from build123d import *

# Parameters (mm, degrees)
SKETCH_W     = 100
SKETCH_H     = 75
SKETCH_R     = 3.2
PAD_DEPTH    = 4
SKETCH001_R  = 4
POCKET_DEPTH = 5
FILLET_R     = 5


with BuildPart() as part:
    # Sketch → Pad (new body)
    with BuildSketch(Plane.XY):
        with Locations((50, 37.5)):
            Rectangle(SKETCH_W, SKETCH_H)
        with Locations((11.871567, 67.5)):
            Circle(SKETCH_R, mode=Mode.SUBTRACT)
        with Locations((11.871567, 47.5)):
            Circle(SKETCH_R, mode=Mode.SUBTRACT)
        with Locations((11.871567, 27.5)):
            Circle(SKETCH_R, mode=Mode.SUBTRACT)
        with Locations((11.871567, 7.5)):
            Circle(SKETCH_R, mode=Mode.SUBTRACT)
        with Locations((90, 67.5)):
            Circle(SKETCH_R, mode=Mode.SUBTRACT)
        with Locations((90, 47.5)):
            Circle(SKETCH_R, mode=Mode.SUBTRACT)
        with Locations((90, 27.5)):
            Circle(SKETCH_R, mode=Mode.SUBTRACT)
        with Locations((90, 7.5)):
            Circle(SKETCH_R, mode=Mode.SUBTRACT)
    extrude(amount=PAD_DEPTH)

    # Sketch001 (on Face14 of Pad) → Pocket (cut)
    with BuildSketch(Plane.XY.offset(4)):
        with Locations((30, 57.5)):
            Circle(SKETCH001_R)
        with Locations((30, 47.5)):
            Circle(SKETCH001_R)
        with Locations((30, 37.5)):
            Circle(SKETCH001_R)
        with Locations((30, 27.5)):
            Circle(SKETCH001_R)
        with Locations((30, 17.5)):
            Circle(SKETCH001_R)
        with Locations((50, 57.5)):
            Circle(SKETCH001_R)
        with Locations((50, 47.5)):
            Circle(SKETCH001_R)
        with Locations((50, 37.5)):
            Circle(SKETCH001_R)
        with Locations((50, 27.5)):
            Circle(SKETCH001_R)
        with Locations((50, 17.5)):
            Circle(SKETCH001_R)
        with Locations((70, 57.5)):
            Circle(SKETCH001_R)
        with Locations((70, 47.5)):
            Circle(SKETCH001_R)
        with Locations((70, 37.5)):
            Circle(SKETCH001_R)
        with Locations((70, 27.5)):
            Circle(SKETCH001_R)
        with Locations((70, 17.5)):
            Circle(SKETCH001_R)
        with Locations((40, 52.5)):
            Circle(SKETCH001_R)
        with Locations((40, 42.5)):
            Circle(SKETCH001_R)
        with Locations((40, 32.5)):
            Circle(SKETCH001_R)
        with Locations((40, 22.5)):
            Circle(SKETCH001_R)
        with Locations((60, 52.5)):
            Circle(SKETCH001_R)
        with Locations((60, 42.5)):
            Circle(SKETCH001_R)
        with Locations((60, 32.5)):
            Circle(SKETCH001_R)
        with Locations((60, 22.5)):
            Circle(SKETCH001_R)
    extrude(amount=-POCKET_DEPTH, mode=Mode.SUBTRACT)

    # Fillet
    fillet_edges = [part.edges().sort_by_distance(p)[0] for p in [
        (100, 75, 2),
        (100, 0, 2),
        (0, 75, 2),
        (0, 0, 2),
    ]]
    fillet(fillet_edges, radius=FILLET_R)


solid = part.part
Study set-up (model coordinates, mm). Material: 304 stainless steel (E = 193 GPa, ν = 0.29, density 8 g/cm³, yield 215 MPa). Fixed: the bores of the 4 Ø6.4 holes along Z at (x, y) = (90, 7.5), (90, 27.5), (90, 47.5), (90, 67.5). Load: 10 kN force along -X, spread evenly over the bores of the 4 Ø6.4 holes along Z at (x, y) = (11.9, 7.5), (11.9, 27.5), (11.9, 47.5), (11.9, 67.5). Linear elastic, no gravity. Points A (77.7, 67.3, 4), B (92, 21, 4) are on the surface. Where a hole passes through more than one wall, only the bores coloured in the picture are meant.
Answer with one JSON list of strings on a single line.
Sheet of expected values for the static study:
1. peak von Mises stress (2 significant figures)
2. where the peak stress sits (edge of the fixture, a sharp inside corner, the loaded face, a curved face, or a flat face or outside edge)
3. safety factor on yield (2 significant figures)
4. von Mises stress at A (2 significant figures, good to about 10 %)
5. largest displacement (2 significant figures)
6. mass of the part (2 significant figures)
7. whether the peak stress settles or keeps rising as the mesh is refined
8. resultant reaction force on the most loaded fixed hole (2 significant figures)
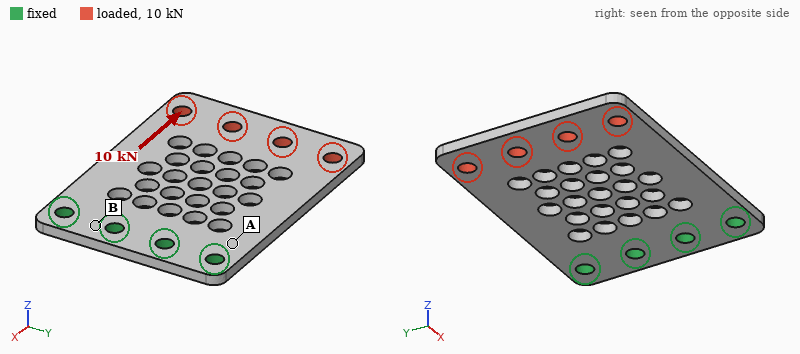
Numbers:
["150 MPa", "a curved face", "1.4", "64 MPa", "28 µm", "190 g", "settles", "3.5 kN"]
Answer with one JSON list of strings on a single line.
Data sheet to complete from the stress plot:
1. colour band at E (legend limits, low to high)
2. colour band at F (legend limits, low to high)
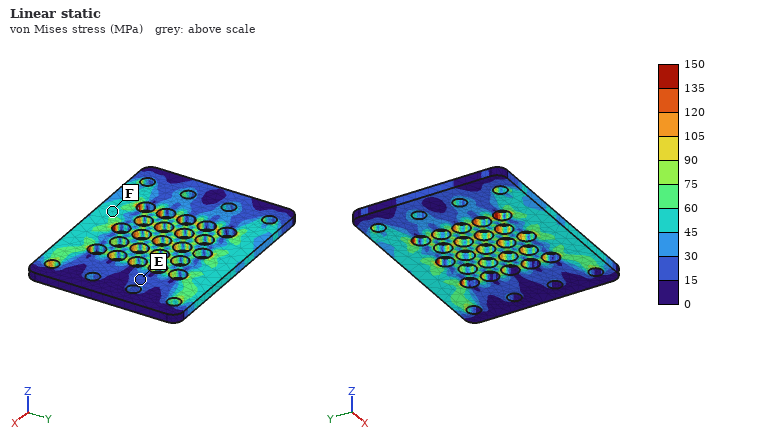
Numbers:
["15 to 30 MPa", "45 to 60 MPa"]
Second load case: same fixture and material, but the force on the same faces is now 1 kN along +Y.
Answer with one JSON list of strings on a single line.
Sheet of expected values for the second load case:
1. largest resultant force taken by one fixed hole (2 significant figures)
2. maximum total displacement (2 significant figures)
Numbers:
["1.2 kN", "23 µm"]
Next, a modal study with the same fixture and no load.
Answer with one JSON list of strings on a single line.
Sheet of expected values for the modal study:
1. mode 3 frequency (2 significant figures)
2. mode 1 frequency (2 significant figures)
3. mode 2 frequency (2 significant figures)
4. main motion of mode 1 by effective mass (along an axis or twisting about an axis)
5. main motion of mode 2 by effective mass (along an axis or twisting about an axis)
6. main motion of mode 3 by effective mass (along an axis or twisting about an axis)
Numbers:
["2300 Hz", "360 Hz", "990 Hz", "along Z", "twisting about X", "along Z"]
